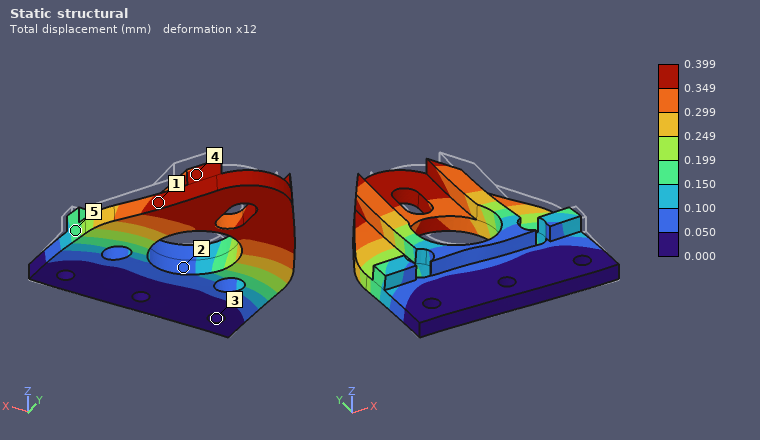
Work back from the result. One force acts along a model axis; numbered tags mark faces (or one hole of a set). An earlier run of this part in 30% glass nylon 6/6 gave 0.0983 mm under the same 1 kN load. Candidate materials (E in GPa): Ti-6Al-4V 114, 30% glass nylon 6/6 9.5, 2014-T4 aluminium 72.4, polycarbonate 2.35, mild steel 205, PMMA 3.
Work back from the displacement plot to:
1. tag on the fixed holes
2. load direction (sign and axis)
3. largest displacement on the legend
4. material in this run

3
-X
0.399 mm
polycarbonate
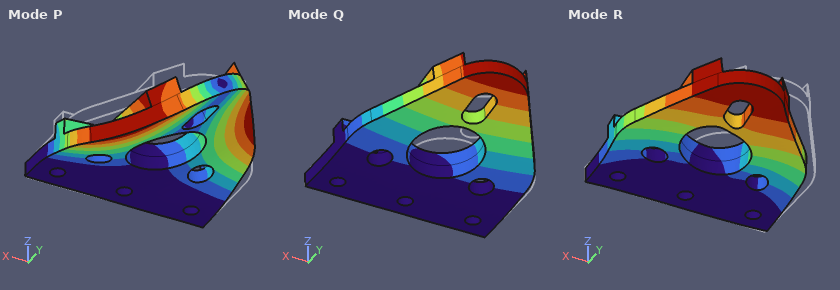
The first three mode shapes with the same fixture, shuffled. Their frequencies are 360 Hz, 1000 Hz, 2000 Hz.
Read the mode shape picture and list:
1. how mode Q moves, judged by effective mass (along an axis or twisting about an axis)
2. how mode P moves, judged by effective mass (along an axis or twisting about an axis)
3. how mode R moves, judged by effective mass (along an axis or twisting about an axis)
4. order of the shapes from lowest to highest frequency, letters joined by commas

along Z
twisting about Y
along X
Q, P, R
